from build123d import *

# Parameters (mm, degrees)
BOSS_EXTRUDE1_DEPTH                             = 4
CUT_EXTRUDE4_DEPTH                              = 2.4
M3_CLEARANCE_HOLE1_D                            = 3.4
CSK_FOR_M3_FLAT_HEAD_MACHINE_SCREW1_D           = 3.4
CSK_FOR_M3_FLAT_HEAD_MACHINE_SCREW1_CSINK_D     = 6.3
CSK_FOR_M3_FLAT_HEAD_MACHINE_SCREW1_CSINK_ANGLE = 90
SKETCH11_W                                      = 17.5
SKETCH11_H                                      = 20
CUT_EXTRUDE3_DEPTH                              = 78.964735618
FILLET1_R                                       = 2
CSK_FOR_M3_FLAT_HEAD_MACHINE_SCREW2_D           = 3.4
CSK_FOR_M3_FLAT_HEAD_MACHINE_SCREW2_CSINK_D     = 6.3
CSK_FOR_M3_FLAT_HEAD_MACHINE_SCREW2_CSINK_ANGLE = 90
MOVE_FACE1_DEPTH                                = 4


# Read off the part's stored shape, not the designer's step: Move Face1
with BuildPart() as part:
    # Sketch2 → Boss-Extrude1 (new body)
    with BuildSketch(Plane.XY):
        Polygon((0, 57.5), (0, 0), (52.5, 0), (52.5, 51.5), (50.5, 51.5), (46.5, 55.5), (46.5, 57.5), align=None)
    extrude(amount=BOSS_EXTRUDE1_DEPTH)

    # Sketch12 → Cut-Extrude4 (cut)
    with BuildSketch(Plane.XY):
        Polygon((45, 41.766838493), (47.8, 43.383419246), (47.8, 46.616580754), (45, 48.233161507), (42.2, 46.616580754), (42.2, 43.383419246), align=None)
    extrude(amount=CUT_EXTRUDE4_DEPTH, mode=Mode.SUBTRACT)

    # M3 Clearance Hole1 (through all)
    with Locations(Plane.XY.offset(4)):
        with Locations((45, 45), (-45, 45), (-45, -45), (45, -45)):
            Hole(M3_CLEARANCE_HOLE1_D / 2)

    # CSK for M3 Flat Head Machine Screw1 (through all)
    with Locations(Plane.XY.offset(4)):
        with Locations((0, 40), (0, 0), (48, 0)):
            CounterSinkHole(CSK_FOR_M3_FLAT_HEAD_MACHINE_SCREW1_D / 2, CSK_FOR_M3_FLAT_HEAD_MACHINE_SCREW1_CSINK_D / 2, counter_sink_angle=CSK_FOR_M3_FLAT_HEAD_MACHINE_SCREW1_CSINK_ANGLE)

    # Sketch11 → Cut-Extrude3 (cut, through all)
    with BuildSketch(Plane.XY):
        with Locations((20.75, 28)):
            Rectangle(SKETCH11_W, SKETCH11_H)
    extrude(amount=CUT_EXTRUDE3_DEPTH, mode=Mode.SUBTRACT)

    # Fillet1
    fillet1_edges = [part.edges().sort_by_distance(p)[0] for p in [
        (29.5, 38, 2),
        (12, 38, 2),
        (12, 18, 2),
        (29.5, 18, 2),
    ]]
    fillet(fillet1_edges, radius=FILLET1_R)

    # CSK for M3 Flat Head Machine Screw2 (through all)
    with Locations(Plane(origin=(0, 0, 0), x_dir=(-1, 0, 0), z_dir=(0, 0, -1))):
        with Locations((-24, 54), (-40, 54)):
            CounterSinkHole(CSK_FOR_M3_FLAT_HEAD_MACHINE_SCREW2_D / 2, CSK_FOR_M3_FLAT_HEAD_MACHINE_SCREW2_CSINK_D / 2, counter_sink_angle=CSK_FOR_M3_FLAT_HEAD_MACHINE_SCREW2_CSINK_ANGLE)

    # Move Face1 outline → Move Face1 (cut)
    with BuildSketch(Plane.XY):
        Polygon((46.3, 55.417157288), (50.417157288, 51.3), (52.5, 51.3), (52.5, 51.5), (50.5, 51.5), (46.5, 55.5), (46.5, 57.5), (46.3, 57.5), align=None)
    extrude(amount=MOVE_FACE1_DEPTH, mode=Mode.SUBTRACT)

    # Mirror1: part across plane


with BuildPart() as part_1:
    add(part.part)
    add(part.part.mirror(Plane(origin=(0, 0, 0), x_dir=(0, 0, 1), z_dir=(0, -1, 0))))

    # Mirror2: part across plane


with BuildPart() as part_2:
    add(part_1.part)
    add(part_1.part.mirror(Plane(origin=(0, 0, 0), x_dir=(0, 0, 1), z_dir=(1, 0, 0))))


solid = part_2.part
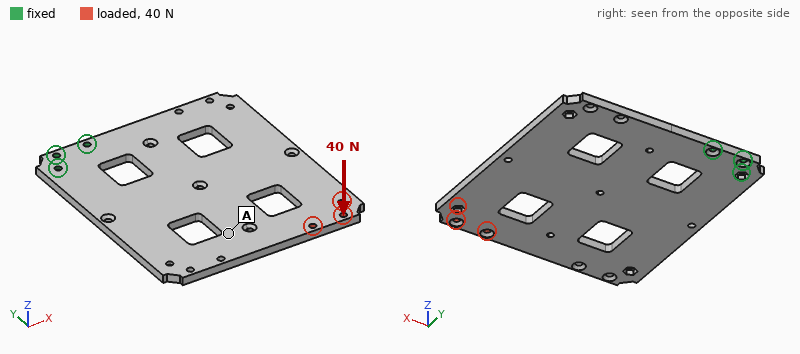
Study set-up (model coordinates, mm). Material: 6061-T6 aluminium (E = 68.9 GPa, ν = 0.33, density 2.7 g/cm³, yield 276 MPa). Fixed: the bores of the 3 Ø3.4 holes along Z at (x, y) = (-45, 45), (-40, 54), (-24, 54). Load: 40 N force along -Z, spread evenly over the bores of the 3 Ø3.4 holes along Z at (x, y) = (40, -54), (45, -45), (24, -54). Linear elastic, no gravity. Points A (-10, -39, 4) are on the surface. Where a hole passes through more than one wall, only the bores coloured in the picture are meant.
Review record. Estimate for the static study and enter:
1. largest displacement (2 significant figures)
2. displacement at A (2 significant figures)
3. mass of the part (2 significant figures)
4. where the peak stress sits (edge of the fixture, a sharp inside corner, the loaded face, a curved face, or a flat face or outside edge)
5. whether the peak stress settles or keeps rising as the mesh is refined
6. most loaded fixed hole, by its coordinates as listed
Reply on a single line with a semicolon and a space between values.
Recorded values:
1.6 mm; 0.85 mm; 110 g; edge of the fixture; keeps rising; (-40, 54)
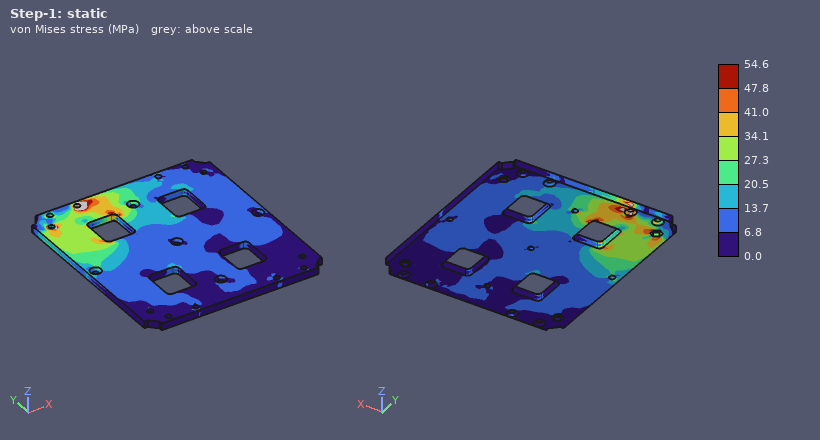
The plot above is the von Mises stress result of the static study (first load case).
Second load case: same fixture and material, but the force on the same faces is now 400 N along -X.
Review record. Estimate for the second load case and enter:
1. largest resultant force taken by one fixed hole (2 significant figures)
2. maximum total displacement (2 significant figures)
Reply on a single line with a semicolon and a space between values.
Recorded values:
1.6 kN; 0.17 mm
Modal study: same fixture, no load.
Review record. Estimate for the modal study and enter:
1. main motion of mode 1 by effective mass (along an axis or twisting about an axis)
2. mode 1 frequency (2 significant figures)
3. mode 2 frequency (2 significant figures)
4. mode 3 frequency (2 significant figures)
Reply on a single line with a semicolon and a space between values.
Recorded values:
along Z; 170 Hz; 390 Hz; 900 Hz
